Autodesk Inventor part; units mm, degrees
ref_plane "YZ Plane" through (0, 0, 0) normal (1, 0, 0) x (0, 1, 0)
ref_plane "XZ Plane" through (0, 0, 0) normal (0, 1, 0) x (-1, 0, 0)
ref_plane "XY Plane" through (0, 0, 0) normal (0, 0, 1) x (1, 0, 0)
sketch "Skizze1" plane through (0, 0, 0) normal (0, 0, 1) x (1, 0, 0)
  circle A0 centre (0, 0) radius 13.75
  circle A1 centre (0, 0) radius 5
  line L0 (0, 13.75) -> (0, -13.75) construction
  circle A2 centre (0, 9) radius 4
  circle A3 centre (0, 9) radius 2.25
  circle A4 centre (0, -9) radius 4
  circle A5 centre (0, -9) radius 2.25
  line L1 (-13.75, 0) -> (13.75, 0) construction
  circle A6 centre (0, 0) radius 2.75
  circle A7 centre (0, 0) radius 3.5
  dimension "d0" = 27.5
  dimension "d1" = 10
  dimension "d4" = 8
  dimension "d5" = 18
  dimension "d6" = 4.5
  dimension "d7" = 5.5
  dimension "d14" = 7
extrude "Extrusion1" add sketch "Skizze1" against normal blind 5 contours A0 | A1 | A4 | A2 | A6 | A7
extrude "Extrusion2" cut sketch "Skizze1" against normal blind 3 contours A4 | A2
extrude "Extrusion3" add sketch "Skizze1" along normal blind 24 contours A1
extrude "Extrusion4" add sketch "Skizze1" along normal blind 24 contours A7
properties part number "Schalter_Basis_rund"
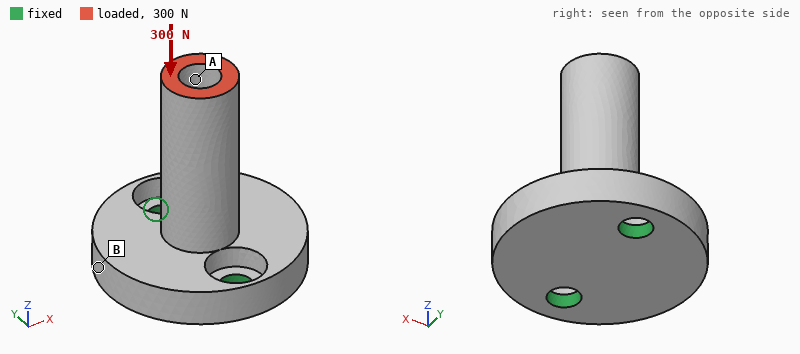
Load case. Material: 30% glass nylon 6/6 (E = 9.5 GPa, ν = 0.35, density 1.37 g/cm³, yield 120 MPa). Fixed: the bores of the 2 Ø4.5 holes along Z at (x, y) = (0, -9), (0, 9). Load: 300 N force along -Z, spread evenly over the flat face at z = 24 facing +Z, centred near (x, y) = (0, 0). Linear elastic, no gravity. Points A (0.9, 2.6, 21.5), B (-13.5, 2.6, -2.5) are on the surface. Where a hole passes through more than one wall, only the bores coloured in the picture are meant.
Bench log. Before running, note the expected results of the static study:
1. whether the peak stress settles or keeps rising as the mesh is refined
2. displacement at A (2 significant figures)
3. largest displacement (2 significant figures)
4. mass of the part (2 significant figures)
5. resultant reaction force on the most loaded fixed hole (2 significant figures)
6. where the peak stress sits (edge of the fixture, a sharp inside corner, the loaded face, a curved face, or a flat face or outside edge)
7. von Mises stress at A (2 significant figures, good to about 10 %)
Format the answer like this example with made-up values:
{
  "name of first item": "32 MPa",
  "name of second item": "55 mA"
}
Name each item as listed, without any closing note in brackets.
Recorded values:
{
  "whether the peak stress settles or keeps rising as the mesh is refined": "keeps rising",
  "displacement at A": "24 µm",
  "largest displacement": "25 µm",
  "mass of the part": "5.4 g",
  "resultant reaction force on the most loaded fixed hole": "160 N",
  "where the peak stress sits": "edge of the fixture",
  "von Mises stress at A": "5.5 MPa"
}
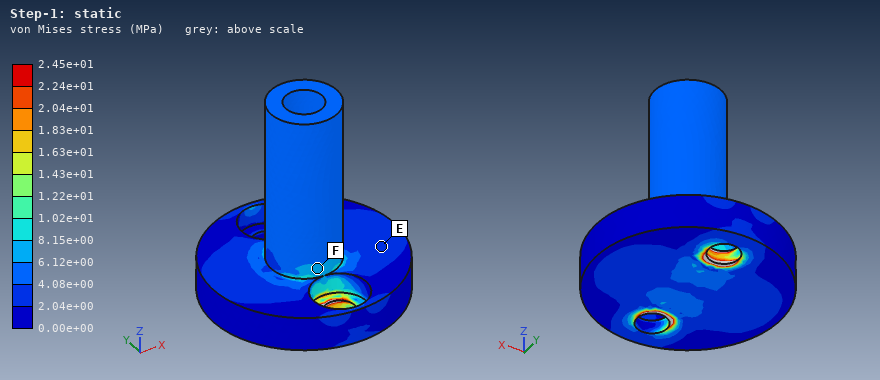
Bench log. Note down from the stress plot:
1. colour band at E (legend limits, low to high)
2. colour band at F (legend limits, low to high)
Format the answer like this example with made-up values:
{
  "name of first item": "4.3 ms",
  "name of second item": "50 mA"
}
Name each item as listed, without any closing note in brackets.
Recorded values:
{
  "colour band at E": "2.04e+00 to 4.08e+00 MPa",
  "colour band at F": "6.12e+00 to 8.15e+00 MPa"
}
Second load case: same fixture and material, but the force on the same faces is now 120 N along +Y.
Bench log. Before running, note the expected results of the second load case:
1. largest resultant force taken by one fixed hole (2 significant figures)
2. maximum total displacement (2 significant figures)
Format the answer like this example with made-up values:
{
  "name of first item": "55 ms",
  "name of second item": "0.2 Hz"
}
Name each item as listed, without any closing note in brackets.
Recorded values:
{
  "largest resultant force taken by one fixed hole": "230 N",
  "maximum total displacement": "0.25 mm"
}
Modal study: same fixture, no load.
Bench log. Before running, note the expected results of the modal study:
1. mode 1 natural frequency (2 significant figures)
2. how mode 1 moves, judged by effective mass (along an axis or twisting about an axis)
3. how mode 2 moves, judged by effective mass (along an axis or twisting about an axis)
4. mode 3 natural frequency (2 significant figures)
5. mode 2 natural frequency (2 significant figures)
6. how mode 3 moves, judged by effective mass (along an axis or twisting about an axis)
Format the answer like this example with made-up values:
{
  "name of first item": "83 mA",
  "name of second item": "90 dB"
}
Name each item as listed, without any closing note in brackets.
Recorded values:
{
  "mode 1 natural frequency": "2900 Hz",
  "how mode 1 moves, judged by effective mass": "along X",
  "how mode 2 moves, judged by effective mass": "along Y",
  "mode 3 natural frequency": "10 kHz",
  "mode 2 natural frequency": "4800 Hz",
  "how mode 3 moves, judged by effective mass": "along Z"
}
